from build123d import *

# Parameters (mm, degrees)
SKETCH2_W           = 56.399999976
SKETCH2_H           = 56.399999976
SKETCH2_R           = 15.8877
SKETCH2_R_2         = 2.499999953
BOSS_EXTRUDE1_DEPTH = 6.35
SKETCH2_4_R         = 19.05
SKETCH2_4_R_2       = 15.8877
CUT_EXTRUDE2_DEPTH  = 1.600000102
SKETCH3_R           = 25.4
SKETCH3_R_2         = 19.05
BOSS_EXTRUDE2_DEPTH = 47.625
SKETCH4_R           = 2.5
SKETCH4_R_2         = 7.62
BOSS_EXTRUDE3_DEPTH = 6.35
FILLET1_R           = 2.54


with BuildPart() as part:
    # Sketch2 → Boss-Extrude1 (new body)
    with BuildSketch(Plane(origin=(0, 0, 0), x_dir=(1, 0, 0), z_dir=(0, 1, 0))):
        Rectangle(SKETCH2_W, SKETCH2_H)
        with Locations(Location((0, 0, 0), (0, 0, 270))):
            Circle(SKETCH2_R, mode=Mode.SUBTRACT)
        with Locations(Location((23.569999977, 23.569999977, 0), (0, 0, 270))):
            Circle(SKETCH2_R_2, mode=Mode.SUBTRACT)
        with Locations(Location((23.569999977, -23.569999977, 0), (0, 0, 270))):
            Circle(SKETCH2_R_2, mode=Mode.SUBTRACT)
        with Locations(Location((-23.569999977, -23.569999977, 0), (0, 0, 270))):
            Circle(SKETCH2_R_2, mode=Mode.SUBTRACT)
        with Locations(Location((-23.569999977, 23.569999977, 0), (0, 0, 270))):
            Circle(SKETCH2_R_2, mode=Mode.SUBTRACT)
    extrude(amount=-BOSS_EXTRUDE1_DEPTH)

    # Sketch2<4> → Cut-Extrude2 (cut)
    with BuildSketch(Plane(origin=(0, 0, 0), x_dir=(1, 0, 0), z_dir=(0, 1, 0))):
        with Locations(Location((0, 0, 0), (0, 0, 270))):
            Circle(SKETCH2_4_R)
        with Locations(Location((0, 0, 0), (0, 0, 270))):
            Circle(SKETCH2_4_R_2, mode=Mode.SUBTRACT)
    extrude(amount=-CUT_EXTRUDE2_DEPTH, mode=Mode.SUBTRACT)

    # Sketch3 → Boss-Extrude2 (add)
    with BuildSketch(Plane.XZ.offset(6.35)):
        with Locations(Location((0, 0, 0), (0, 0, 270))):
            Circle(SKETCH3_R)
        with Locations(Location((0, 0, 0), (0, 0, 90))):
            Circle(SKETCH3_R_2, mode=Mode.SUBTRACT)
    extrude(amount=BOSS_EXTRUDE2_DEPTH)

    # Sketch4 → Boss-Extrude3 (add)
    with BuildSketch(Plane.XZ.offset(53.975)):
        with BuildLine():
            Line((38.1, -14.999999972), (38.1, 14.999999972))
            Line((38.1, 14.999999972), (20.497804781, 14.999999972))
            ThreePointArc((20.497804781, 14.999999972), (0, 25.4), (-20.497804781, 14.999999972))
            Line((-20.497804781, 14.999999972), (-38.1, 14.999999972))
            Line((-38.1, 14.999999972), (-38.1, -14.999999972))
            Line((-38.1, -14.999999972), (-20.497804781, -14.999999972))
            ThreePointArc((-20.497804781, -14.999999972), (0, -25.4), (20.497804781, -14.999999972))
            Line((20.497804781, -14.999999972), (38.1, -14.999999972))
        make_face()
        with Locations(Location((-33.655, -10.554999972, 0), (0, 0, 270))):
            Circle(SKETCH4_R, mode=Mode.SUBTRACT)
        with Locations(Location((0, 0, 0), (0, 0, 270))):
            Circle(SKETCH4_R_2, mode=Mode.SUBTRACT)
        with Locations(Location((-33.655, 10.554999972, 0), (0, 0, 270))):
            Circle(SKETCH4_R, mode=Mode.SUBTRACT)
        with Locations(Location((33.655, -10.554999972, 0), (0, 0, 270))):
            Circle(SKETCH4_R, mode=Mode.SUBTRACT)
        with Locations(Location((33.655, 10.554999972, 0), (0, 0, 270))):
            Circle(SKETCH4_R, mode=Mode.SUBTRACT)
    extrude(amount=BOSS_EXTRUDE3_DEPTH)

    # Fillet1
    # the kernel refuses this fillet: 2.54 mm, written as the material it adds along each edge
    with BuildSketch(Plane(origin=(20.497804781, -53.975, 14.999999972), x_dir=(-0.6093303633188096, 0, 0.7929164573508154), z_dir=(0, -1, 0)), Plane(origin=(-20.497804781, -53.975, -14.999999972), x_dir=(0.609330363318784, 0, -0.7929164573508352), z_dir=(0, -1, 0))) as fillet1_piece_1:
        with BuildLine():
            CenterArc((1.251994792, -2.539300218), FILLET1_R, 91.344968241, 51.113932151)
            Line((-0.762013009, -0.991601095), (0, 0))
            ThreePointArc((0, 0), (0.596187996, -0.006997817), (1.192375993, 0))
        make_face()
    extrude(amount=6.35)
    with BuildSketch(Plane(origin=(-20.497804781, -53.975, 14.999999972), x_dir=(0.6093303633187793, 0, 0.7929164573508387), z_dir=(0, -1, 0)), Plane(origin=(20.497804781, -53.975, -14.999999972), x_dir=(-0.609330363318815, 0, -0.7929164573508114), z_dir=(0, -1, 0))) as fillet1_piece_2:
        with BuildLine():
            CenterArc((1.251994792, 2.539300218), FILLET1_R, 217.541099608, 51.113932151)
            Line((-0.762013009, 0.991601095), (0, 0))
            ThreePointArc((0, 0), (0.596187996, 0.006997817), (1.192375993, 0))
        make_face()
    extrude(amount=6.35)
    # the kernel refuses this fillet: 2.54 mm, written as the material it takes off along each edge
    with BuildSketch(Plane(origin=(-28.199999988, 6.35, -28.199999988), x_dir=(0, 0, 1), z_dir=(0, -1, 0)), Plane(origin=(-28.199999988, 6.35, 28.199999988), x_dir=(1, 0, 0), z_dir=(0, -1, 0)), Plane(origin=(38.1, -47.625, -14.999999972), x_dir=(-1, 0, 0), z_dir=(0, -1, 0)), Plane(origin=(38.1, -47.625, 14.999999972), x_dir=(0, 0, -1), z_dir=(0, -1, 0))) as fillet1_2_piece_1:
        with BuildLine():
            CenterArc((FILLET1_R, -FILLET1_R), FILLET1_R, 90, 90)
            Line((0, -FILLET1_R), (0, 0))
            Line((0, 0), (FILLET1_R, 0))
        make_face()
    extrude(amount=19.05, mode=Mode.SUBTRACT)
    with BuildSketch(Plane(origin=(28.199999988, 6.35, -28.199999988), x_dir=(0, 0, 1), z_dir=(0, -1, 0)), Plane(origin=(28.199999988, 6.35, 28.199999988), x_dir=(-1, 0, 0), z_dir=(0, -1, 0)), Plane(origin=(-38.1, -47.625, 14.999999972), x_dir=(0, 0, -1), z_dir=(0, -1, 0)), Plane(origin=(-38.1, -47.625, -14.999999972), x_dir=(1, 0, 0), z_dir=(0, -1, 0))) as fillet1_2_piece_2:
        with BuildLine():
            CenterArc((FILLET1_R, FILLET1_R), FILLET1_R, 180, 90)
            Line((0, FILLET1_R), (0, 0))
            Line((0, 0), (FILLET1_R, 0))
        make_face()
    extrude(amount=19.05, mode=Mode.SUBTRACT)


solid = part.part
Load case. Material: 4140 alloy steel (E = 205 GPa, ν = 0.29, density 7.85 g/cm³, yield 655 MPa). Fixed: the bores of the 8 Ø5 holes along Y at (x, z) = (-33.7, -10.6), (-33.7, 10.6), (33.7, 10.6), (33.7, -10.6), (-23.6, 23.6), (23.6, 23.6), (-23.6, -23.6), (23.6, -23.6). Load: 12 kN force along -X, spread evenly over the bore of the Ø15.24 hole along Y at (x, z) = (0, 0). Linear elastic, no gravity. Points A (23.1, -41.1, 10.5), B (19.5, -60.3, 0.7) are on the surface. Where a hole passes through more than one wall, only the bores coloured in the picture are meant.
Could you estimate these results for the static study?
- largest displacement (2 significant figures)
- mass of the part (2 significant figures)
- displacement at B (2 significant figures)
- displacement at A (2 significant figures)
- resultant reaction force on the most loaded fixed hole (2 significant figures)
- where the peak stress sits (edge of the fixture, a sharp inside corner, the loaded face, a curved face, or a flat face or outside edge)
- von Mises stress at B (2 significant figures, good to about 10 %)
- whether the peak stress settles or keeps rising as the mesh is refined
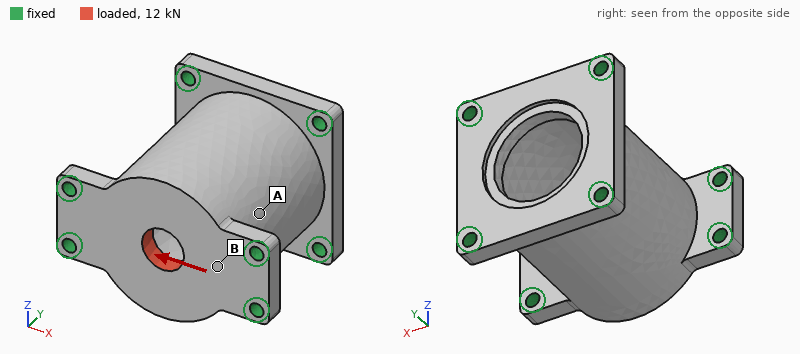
5.3 µm
570 g
2.5 µm
1.8 µm
2.9 kN
edge of the fixture
32 MPa
keeps rising
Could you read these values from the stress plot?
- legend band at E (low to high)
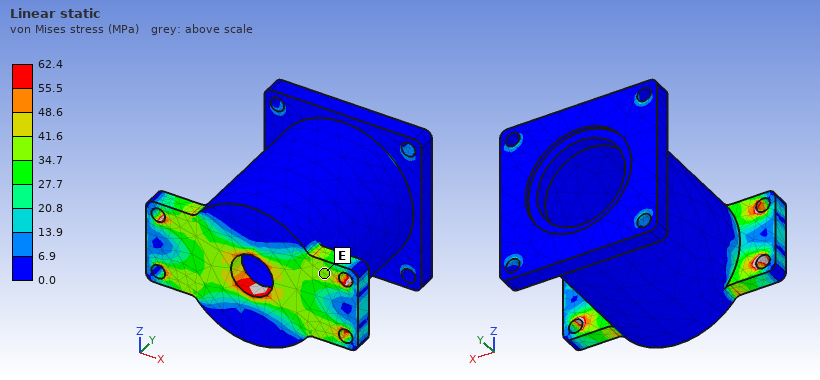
34.7 to 41.6 MPa
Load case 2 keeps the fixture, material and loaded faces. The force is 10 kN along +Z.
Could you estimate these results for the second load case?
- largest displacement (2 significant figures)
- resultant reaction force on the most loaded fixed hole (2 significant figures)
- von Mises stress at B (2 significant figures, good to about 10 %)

10 µm
3.0 kN
38 MPa
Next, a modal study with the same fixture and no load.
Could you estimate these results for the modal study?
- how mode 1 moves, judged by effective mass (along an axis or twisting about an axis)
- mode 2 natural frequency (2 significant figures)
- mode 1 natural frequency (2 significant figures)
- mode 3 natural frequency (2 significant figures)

along Y
13 kHz
9600 Hz
13 kHz
